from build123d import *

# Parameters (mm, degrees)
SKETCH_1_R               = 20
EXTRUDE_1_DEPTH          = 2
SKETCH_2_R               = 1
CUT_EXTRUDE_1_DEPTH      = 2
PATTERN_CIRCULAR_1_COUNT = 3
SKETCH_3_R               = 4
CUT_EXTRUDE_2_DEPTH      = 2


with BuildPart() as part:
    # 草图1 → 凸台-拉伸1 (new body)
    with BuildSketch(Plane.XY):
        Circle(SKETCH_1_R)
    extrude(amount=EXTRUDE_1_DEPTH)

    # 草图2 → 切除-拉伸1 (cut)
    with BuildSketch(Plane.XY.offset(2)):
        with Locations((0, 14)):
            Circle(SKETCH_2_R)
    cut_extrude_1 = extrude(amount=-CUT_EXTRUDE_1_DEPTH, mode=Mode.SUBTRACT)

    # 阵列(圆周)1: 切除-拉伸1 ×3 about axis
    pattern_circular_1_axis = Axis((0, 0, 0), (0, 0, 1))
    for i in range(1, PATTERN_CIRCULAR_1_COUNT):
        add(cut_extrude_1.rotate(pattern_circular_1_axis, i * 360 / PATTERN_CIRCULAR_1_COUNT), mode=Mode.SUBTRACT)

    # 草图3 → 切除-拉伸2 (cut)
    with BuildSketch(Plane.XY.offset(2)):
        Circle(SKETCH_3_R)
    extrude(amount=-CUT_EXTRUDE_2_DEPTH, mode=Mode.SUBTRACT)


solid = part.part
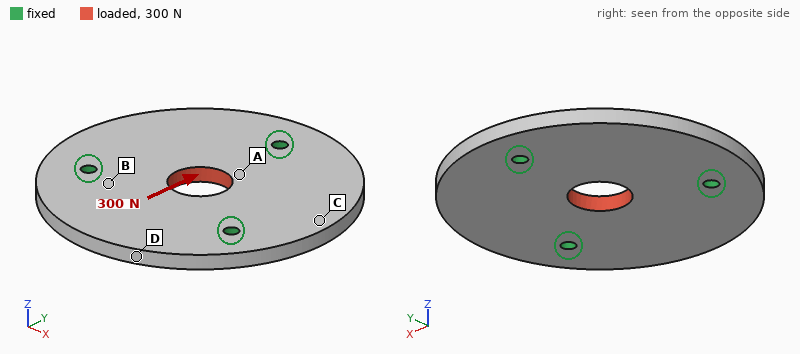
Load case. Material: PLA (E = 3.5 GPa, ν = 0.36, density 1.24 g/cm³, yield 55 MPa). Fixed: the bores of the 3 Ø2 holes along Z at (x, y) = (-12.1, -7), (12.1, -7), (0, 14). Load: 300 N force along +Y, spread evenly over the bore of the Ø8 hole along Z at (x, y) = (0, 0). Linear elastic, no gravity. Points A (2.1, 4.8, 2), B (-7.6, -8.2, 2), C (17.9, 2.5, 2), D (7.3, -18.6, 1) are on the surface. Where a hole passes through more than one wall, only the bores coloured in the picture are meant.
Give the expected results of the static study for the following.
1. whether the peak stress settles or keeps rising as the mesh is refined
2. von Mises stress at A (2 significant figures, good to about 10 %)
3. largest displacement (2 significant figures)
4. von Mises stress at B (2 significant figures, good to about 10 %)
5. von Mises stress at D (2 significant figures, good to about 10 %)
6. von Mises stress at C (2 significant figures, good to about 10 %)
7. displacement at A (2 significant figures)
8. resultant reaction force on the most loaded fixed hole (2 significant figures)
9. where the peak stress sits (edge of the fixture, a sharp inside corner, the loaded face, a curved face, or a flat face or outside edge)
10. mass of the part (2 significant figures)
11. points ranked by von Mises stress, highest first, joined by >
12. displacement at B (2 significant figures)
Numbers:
keeps rising
7.1 MPa
29 µm
3.8 MPa
2.6 MPa
1.1 MPa
18 µm
100 N
edge of the fixture
3.0 g
A > B > D > C
13 µm
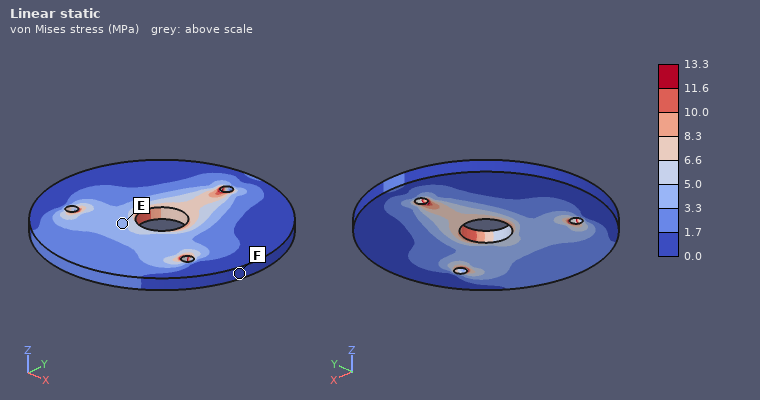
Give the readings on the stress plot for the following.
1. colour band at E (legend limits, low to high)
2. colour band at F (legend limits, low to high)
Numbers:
3.3 to 5.0 MPa
0.0 to 1.7 MPa
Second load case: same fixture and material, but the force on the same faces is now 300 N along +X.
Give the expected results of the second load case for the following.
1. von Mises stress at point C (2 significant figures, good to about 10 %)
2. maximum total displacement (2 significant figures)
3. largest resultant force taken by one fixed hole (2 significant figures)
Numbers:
2.2 MPa
29 µm
100 N
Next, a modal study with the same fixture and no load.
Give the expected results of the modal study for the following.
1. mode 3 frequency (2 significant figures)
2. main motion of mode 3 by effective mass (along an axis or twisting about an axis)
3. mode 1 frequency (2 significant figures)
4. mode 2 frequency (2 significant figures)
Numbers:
3300 Hz
along Z
2900 Hz
2900 Hz
